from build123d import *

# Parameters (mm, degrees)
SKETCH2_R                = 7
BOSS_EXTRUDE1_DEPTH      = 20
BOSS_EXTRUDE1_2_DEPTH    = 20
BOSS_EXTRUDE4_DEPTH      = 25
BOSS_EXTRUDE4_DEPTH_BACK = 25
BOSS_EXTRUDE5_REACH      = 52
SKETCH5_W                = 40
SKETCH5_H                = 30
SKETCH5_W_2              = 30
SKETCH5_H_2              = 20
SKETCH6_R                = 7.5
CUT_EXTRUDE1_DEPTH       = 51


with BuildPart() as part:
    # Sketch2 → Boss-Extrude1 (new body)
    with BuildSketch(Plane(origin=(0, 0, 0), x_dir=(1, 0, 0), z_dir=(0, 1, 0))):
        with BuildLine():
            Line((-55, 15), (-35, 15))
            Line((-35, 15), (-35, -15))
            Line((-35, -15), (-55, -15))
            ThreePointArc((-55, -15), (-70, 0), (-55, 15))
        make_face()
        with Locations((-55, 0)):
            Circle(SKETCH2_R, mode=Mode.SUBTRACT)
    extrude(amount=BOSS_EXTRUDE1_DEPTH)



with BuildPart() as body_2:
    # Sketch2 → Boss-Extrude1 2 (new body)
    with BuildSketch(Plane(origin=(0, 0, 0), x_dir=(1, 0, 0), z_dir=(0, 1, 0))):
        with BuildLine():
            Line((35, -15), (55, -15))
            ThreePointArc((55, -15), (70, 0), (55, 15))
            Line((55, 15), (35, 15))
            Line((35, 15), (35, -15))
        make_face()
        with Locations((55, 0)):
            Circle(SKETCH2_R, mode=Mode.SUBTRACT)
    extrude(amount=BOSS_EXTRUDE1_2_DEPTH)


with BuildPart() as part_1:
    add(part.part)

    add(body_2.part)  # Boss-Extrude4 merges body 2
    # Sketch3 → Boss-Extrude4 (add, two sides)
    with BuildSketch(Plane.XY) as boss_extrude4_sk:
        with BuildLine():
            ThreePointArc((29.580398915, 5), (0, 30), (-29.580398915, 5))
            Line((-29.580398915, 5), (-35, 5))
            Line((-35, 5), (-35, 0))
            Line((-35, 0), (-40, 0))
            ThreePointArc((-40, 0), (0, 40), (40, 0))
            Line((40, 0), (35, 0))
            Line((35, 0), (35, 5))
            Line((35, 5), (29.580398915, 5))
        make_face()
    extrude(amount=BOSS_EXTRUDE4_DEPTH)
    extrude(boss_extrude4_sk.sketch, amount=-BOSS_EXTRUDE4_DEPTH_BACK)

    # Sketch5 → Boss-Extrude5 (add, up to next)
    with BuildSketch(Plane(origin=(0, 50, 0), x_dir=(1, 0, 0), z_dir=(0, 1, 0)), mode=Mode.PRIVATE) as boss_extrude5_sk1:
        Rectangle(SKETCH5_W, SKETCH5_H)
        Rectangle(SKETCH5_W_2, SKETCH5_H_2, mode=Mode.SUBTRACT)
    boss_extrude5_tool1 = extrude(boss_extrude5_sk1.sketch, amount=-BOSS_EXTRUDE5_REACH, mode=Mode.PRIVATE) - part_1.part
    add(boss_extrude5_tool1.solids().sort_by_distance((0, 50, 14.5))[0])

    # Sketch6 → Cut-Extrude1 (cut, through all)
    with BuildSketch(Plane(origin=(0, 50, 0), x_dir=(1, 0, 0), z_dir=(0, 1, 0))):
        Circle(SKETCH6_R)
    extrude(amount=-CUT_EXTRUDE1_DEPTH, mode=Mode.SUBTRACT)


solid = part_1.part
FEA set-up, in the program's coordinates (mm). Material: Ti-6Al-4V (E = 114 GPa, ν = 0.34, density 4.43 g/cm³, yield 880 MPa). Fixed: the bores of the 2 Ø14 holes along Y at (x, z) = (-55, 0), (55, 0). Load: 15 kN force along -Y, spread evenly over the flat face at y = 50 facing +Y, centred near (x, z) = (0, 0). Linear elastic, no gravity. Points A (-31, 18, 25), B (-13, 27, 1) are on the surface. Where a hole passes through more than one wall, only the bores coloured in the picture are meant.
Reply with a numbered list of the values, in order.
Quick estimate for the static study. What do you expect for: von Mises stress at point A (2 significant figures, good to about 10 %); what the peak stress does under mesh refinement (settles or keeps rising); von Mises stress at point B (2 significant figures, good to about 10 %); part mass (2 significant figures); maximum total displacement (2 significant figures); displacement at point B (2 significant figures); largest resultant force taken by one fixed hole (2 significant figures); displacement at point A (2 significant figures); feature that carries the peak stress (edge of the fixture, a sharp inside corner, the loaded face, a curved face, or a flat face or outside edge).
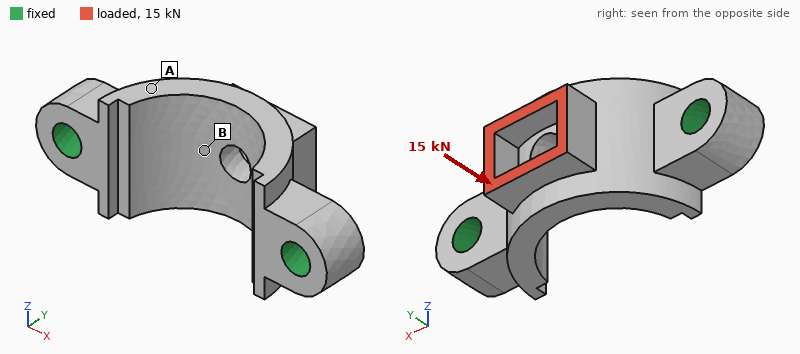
1. 6.7 MPa
2. keeps rising
3. 12 MPa
4. 380 g
5. 24 µm
6. 21 µm
7. 10 kN
8. 12 µm
9. edge of the fixture
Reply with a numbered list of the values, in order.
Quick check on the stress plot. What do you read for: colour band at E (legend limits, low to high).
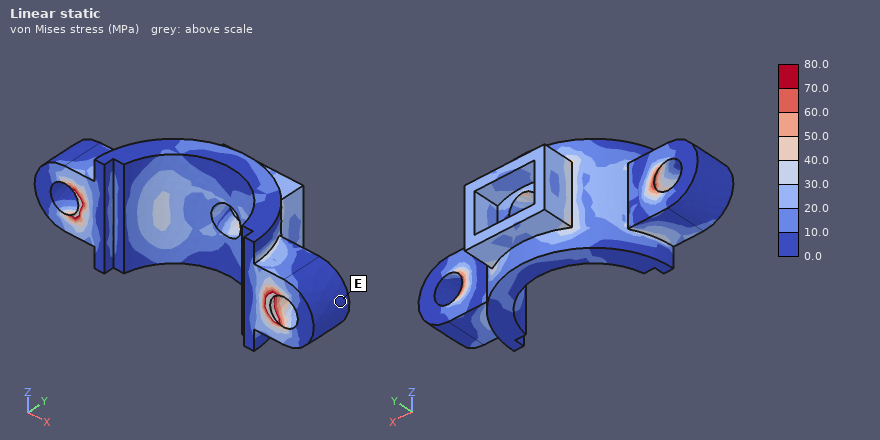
1. 0.0 to 10.0 MPa
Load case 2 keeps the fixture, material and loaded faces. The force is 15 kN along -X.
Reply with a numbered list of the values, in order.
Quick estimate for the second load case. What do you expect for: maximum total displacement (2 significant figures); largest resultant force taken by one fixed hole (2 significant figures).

1. 62 µm
2. 11 kN
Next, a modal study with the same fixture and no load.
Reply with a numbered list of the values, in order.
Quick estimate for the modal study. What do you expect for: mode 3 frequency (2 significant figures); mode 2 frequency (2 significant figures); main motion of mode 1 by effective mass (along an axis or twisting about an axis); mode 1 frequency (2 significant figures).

1. 10 kHz
2. 10000 Hz
3. along Z
4. 4700 Hz
